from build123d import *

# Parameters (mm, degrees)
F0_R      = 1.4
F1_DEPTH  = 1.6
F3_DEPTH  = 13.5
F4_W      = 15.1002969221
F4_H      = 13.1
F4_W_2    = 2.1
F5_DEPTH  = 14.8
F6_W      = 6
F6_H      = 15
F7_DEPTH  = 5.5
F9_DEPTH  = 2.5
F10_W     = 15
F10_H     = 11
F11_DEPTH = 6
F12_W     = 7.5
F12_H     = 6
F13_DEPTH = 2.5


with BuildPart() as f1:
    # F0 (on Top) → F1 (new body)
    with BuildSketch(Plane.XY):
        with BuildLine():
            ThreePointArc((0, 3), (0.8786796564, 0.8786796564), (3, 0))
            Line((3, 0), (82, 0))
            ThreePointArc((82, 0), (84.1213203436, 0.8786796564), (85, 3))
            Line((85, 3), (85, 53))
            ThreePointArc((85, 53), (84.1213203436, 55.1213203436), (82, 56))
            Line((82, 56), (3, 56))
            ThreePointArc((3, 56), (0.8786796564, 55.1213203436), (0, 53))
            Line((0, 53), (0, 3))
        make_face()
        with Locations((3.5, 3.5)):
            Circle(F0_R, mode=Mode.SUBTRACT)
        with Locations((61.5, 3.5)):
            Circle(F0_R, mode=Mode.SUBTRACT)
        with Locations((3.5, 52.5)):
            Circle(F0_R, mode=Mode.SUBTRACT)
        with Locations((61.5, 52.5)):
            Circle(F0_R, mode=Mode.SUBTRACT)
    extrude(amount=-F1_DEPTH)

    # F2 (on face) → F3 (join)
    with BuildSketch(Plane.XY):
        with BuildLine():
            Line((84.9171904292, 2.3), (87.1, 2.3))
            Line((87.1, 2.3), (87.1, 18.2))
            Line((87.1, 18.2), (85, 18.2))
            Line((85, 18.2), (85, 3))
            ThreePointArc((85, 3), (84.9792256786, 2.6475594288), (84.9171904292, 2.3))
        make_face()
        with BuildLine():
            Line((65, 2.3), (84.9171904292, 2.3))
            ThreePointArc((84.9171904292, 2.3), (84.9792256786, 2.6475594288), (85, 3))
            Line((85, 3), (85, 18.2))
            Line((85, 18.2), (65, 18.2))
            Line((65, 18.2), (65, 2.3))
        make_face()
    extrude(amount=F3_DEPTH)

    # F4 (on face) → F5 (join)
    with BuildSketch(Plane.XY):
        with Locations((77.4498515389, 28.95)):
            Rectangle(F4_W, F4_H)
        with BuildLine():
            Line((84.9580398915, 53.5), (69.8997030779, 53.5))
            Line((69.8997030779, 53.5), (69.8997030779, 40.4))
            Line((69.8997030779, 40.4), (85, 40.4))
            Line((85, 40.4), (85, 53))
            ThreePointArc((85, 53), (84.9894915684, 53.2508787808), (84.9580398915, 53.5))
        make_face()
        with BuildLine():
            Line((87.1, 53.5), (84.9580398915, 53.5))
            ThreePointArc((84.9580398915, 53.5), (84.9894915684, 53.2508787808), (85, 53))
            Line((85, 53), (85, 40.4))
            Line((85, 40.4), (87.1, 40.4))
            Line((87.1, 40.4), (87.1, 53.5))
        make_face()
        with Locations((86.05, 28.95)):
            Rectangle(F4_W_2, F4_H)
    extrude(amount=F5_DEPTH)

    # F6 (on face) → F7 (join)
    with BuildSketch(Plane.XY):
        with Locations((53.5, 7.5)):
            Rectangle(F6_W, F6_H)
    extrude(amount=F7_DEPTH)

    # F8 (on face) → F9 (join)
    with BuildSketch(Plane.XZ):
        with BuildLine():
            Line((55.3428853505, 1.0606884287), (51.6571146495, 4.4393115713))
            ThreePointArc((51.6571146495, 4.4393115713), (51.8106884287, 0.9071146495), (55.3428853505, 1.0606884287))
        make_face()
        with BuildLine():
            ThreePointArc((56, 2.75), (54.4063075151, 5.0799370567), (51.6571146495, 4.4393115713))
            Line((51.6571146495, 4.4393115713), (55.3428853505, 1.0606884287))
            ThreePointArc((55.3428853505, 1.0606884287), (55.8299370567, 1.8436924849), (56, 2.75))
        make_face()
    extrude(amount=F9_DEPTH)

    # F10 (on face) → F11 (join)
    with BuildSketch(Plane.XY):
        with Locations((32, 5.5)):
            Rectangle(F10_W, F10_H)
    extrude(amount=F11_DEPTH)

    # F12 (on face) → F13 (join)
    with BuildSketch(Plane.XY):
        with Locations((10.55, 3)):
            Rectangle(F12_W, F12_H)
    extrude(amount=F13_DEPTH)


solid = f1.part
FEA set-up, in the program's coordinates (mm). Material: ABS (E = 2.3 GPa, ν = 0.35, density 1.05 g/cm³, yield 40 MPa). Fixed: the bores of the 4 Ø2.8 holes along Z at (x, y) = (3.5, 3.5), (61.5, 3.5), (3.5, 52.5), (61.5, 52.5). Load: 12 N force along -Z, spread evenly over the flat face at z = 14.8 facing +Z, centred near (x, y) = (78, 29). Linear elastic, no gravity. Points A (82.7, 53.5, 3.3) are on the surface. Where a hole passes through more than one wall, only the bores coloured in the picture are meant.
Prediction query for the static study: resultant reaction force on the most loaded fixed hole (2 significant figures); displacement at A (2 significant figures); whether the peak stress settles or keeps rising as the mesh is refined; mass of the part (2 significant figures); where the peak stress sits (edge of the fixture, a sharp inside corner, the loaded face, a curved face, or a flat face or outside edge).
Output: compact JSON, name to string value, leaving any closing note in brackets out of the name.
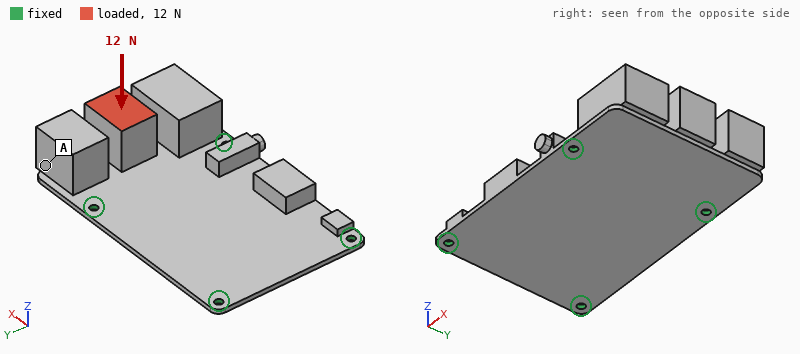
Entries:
{"resultant reaction force on the most loaded fixed hole": "6.7 N", "displacement at A": "0.62 mm", "whether the peak stress settles or keeps rising as the mesh is refined": "keeps rising", "mass of the part": "22 g", "where the peak stress sits": "edge of the fixture"}
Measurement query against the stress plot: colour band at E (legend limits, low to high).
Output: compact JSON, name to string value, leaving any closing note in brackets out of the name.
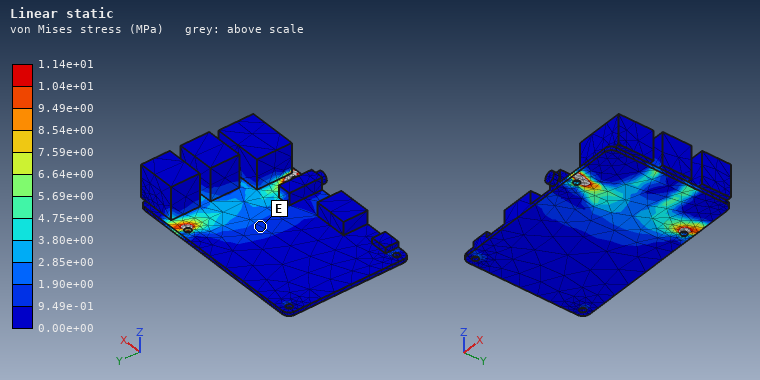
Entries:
{"colour band at E": "9.49e-01 to 1.90e+00 MPa"}
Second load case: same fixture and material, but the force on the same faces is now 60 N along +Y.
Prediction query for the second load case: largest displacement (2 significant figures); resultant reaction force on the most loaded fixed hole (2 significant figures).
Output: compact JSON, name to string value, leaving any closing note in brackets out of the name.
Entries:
{"largest displacement": "1.1 mm", "resultant reaction force on the most loaded fixed hole": "44 N"}
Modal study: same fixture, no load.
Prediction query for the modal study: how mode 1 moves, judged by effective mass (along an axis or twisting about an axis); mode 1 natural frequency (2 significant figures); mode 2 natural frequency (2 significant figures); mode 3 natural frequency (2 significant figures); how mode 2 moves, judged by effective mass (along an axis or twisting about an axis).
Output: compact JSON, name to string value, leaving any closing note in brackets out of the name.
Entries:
{"how mode 1 moves, judged by effective mass": "along Z", "mode 1 natural frequency": "180 Hz", "mode 2 natural frequency": "530 Hz", "mode 3 natural frequency": "610 Hz", "how mode 2 moves, judged by effective mass": "along Z"}
